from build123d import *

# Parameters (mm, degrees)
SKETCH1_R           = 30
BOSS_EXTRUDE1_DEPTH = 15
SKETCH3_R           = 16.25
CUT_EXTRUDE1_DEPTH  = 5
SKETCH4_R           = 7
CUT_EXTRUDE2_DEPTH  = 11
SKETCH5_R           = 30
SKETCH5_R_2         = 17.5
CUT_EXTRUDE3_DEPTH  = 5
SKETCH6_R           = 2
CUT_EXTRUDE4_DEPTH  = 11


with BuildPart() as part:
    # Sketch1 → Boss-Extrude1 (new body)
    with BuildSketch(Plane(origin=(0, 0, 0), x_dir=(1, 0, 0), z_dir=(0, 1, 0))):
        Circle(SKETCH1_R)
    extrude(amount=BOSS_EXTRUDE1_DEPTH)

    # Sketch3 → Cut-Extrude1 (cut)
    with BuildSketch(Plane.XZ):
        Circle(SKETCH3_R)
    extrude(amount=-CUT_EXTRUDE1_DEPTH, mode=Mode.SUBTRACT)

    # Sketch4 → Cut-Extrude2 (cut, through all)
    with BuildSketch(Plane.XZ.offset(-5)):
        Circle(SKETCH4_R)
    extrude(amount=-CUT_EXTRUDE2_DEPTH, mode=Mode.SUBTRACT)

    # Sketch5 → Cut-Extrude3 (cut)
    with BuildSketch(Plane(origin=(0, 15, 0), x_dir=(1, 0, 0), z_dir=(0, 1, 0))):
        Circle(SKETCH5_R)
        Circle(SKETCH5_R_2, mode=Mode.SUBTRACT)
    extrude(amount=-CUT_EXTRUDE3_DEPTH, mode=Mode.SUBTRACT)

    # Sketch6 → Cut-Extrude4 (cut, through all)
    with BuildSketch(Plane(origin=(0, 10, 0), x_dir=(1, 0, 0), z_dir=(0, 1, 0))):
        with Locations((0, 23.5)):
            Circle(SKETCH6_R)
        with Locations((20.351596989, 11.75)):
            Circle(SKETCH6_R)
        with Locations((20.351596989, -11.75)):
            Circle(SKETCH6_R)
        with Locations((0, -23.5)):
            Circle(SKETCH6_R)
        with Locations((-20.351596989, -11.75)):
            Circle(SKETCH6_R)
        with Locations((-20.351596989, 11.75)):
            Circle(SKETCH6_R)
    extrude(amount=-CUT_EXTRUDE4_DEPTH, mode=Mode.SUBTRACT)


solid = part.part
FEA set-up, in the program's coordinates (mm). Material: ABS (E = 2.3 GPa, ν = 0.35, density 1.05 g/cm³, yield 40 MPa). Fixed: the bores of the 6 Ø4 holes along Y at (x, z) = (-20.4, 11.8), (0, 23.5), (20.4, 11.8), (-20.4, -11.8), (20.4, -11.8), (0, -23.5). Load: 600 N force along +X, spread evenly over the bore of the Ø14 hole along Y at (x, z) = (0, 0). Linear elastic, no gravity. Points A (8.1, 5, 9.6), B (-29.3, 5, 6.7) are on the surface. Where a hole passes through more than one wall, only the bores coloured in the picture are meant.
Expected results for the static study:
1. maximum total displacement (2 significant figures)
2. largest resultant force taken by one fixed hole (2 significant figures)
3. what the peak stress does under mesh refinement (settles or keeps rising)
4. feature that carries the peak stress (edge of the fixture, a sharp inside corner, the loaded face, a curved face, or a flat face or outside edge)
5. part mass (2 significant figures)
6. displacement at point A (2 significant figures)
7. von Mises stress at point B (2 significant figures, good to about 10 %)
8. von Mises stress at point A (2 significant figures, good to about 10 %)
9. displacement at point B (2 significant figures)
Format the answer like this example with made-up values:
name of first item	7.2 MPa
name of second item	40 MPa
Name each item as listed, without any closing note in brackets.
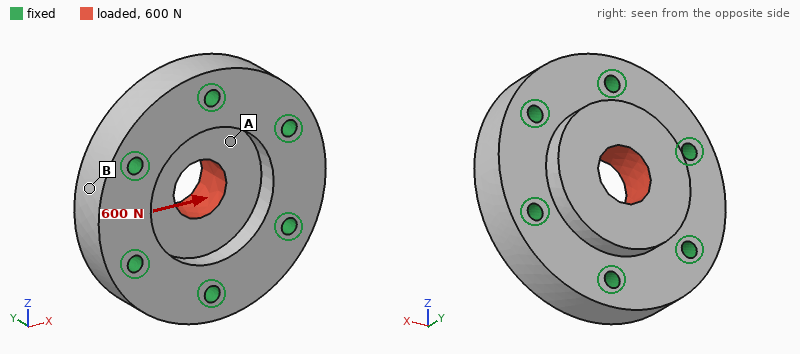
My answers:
maximum total displacement	17 µm
largest resultant force taken by one fixed hole	130 N
what the peak stress does under mesh refinement	keeps rising
feature that carries the peak stress	edge of the fixture
part mass	28 g
displacement at point A	6.7 µm
von Mises stress at point B	0.45 MPa
von Mises stress at point A	1.6 MPa
displacement at point B	3.5 µm
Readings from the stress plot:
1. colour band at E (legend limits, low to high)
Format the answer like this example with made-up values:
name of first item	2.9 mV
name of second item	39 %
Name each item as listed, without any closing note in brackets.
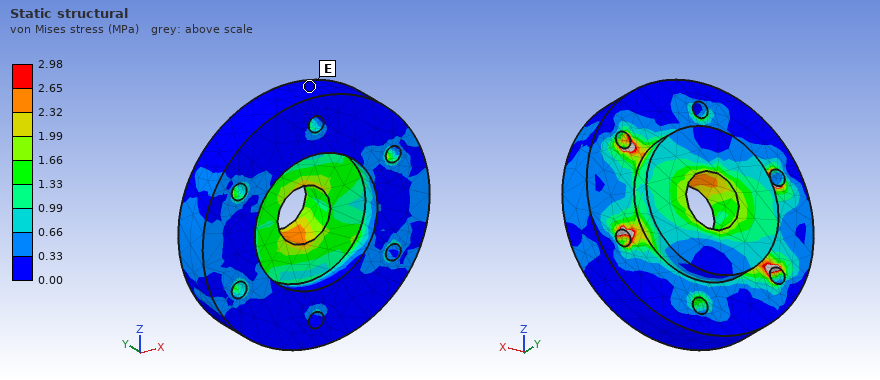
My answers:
colour band at E	0.00 to 0.33 MPa
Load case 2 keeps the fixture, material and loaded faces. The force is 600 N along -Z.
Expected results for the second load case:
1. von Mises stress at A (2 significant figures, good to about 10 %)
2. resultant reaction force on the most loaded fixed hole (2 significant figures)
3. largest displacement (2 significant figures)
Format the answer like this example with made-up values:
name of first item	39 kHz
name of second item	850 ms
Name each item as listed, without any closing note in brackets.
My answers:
von Mises stress at A	1.2 MPa
resultant reaction force on the most loaded fixed hole	150 N
largest displacement	17 µm
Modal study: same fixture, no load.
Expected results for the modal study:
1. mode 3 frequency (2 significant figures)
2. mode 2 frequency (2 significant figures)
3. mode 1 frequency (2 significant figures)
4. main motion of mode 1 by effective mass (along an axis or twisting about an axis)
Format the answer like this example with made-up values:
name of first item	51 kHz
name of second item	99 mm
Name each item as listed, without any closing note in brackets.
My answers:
mode 3 frequency	12 kHz
mode 2 frequency	12 kHz
mode 1 frequency	9300 Hz
main motion of mode 1 by effective mass	along Y
